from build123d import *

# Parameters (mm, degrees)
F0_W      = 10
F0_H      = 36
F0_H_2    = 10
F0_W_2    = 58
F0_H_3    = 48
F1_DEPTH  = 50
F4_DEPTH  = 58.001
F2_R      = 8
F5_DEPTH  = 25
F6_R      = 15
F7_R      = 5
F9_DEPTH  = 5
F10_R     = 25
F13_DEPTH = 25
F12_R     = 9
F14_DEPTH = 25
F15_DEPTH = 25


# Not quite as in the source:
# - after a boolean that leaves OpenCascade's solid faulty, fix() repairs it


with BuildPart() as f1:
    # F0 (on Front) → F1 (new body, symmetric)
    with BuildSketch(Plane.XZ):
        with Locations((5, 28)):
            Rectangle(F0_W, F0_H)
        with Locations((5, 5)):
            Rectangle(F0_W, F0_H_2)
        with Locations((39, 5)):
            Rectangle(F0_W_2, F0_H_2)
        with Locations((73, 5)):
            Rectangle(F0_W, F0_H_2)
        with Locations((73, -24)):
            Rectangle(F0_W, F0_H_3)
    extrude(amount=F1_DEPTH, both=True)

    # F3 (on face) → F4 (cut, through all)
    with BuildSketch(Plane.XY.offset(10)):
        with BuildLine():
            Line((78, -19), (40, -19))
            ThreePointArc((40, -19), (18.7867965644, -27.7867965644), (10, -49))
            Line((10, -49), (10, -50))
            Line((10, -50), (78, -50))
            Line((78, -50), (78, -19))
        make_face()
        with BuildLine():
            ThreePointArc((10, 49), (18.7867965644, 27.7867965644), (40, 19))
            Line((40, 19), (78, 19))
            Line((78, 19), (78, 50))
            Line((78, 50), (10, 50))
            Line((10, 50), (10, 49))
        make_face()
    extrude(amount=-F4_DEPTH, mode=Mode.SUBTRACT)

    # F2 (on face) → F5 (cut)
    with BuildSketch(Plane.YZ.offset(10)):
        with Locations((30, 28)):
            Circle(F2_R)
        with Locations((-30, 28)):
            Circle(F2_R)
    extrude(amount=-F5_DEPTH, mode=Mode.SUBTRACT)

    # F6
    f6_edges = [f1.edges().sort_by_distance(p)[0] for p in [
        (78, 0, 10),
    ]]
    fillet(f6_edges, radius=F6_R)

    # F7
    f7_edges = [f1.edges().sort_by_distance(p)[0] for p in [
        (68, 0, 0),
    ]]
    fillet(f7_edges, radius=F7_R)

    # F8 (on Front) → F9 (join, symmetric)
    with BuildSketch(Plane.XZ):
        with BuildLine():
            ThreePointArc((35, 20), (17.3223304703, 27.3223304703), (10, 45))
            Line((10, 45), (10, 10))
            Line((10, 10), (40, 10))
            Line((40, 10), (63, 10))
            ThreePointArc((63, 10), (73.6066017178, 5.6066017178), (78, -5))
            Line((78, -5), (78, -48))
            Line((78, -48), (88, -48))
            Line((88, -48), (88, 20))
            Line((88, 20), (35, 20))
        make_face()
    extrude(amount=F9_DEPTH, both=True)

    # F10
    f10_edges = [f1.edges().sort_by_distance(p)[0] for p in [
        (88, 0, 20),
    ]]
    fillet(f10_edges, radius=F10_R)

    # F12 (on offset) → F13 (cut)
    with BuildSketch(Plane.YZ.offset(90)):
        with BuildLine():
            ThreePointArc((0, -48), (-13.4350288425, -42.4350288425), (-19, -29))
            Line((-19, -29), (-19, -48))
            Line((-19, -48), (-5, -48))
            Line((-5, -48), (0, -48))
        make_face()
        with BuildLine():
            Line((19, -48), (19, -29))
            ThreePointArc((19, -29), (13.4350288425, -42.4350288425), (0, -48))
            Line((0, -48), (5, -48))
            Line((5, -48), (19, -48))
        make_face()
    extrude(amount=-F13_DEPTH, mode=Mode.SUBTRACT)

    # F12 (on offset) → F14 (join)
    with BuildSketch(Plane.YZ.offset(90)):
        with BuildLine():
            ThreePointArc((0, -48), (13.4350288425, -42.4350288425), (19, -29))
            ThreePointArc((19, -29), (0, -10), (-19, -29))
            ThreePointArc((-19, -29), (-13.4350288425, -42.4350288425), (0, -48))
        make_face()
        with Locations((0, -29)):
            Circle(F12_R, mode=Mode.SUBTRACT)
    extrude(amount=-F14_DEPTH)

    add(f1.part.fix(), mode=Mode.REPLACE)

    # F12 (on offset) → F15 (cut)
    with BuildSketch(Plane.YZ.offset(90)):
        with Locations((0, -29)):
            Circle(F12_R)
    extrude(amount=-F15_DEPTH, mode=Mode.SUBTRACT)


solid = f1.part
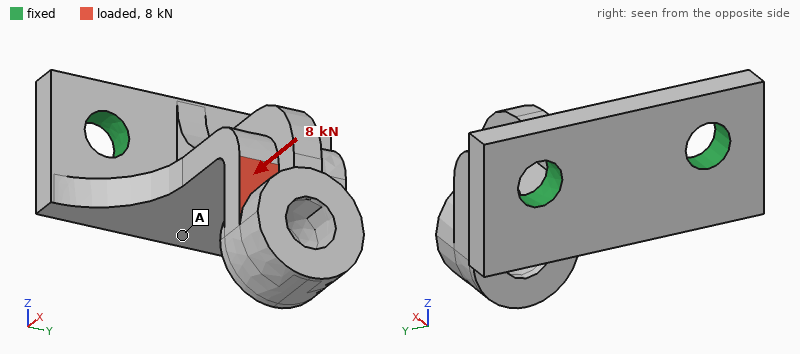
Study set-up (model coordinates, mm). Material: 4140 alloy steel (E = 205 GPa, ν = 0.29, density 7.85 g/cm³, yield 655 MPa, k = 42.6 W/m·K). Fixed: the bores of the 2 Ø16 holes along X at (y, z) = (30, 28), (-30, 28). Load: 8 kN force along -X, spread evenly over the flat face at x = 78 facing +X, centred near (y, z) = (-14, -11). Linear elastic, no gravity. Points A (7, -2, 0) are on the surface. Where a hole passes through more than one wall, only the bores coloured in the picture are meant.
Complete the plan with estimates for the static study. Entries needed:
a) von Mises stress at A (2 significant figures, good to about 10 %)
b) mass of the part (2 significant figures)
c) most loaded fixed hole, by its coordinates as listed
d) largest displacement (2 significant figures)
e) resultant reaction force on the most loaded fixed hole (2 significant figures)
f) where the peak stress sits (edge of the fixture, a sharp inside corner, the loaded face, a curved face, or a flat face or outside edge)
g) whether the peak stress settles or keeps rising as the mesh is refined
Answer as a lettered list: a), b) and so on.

a) 27 MPa
b) 850 g
c) (-30, 28)
d) 0.42 mm
e) 6.1 kN
f) edge of the fixture
g) keeps rising
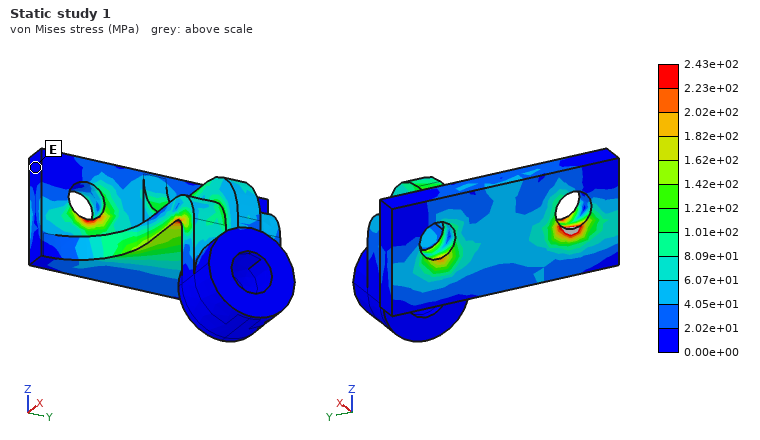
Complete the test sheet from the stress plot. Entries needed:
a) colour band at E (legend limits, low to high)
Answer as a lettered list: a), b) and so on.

a) 0.00e+00 to 2.02e+01 MPa
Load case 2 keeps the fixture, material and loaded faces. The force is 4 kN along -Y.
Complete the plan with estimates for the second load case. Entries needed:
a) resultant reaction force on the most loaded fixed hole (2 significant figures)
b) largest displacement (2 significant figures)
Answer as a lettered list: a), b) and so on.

a) 5.8 kN
b) 0.19 mm
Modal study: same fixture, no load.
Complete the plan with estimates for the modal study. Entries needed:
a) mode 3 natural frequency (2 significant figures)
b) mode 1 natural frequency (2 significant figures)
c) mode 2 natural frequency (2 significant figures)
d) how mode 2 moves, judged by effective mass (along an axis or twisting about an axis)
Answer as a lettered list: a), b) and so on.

a) 3100 Hz
b) 980 Hz
c) 1400 Hz
d) along Y
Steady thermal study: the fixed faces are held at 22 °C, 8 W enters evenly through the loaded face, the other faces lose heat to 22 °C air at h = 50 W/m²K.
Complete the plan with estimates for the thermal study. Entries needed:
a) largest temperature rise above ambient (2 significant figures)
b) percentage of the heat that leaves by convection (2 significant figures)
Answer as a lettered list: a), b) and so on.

a) 20 K
b) 75 %
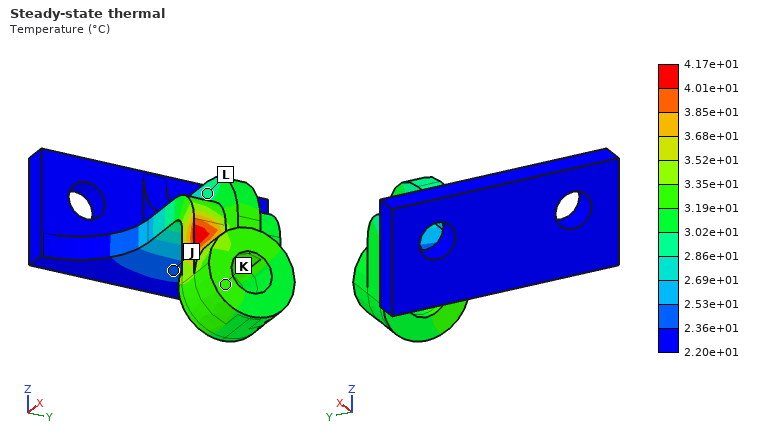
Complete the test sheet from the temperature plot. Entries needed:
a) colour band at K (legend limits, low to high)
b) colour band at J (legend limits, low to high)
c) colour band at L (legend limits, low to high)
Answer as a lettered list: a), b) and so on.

a) 3.19e+01 to 3.35e+01 °C
b) 2.36e+01 to 2.53e+01 °C
c) 2.86e+01 to 3.02e+01 °C
